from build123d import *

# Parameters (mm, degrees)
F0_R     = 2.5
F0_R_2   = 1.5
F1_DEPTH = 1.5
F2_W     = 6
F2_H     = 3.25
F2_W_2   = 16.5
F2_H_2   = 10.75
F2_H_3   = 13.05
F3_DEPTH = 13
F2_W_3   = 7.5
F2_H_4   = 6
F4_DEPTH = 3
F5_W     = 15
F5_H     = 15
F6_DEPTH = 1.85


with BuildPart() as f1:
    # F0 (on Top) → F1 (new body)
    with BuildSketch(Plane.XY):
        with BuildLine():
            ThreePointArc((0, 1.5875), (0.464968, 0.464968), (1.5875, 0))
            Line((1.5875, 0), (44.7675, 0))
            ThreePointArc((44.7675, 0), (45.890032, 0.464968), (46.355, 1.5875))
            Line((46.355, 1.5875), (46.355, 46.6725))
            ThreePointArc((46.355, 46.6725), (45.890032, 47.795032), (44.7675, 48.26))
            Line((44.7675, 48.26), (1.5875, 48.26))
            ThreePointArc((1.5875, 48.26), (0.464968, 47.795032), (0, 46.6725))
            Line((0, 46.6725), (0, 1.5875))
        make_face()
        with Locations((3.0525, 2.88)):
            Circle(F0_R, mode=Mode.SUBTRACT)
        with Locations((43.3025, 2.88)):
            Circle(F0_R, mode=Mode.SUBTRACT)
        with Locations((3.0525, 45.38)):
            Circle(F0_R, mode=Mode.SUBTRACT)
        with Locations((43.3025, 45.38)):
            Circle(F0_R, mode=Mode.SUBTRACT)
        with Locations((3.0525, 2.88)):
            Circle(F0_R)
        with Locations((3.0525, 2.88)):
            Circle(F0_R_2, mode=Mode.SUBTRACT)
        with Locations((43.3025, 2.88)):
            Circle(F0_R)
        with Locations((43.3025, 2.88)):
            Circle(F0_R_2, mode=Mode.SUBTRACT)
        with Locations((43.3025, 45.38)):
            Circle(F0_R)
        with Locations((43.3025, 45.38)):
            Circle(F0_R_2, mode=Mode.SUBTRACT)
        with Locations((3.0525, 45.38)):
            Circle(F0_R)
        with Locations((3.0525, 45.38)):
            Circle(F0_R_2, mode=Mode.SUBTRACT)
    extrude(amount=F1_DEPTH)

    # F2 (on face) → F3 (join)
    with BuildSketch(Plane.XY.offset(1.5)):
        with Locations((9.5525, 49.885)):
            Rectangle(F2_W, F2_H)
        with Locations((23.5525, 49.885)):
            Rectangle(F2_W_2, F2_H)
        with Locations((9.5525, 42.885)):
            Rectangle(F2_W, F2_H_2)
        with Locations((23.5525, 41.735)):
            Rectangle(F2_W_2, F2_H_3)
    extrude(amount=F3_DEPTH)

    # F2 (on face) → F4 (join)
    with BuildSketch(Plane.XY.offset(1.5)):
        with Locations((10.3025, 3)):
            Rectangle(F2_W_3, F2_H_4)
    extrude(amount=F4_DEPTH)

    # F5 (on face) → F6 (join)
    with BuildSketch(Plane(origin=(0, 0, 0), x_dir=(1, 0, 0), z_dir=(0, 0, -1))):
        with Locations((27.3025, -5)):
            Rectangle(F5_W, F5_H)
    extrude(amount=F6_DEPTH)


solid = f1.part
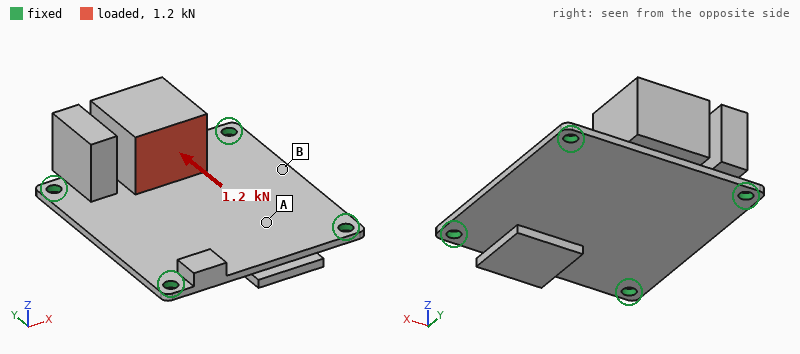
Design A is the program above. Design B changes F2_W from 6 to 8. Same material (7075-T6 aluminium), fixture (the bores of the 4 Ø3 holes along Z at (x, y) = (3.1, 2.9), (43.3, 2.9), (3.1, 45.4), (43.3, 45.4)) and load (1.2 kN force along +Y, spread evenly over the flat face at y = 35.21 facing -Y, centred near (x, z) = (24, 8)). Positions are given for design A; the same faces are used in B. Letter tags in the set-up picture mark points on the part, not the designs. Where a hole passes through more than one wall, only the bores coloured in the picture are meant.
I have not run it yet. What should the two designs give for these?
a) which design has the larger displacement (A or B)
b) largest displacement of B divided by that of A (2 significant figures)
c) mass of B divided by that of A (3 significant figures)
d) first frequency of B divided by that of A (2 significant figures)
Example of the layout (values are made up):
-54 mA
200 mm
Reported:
A
0.85
1.04
1.0
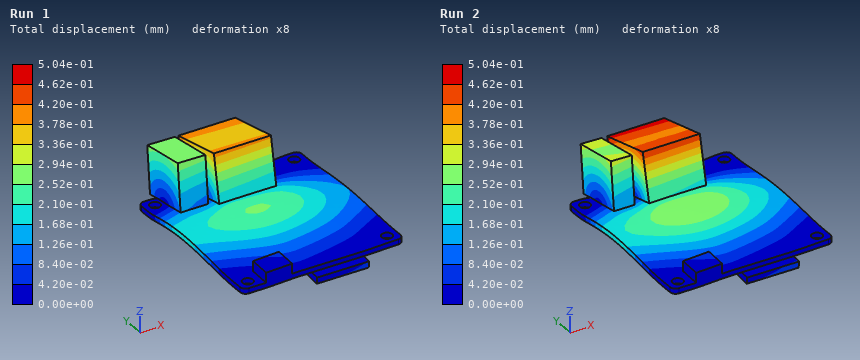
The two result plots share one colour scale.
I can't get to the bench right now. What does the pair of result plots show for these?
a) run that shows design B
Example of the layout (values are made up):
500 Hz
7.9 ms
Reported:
Run 1
